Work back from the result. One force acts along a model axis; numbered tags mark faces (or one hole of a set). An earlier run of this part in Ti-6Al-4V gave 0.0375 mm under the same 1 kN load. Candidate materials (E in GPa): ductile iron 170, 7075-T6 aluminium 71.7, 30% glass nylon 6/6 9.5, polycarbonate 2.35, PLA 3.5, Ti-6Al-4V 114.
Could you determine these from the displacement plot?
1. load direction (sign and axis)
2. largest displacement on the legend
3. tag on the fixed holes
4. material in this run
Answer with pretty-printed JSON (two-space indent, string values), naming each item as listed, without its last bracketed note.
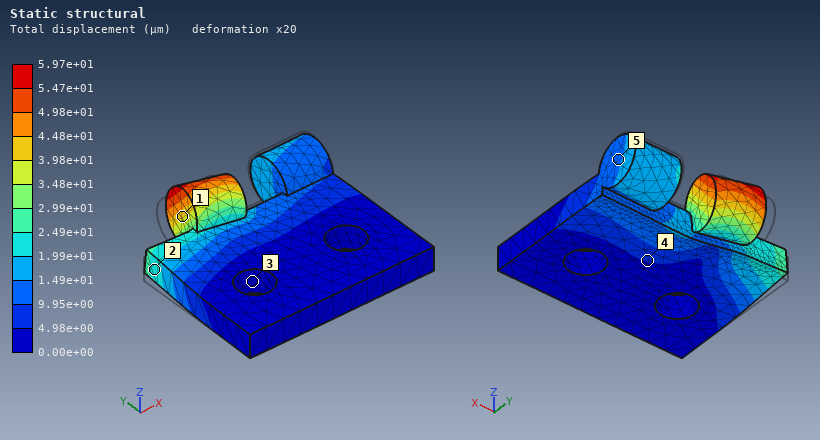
{
  "load direction": "+X",
  "largest displacement on the legend": "5.97e+01 µm",
  "tag on the fixed holes": "3",
  "material in this run": "7075-T6 aluminium"
}
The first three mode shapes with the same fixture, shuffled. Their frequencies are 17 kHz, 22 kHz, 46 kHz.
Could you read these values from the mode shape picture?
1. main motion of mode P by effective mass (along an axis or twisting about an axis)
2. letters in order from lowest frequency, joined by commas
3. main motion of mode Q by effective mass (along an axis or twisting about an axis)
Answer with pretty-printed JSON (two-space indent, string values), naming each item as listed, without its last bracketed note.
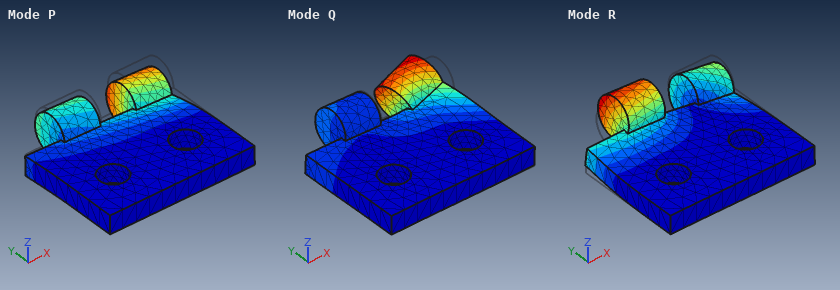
{
  "main motion of mode P by effective mass": "along Z",
  "letters in order from lowest frequency, joined by commas": "P, R, Q",
  "main motion of mode Q by effective mass": "along X"
}
